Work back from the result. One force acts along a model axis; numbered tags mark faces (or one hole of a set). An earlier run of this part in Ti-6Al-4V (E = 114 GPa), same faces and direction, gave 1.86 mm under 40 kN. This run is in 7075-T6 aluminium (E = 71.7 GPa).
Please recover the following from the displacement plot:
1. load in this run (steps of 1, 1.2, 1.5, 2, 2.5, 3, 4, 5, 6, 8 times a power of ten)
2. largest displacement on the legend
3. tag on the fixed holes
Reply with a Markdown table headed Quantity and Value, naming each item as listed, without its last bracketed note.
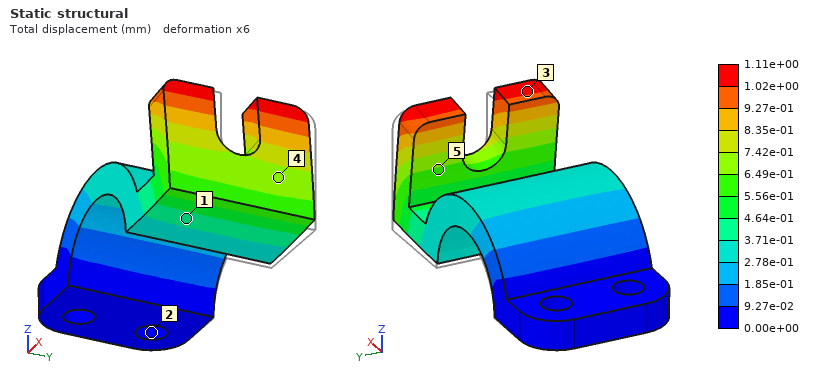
| Quantity | Value |
|---|---|
| load in this run | 15 kN |
| largest displacement on the legend | 1.11e+00 mm |
| tag on the fixed holes | 2 |
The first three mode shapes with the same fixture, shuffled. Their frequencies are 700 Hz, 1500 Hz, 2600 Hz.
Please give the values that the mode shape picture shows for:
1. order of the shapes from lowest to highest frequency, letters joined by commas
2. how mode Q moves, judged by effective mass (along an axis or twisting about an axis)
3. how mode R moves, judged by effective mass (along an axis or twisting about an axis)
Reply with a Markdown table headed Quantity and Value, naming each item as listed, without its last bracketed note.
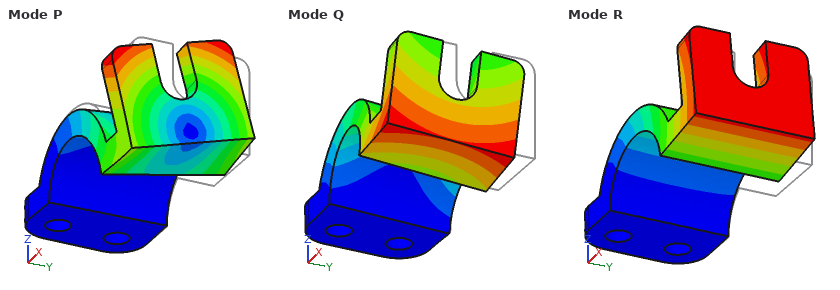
| Quantity | Value |
|---|---|
| order of the shapes from lowest to highest frequency, letters joined by commas | R, Q, P |
| how mode Q moves, judged by effective mass | along Y |
| how mode R moves, judged by effective mass | along Z |
